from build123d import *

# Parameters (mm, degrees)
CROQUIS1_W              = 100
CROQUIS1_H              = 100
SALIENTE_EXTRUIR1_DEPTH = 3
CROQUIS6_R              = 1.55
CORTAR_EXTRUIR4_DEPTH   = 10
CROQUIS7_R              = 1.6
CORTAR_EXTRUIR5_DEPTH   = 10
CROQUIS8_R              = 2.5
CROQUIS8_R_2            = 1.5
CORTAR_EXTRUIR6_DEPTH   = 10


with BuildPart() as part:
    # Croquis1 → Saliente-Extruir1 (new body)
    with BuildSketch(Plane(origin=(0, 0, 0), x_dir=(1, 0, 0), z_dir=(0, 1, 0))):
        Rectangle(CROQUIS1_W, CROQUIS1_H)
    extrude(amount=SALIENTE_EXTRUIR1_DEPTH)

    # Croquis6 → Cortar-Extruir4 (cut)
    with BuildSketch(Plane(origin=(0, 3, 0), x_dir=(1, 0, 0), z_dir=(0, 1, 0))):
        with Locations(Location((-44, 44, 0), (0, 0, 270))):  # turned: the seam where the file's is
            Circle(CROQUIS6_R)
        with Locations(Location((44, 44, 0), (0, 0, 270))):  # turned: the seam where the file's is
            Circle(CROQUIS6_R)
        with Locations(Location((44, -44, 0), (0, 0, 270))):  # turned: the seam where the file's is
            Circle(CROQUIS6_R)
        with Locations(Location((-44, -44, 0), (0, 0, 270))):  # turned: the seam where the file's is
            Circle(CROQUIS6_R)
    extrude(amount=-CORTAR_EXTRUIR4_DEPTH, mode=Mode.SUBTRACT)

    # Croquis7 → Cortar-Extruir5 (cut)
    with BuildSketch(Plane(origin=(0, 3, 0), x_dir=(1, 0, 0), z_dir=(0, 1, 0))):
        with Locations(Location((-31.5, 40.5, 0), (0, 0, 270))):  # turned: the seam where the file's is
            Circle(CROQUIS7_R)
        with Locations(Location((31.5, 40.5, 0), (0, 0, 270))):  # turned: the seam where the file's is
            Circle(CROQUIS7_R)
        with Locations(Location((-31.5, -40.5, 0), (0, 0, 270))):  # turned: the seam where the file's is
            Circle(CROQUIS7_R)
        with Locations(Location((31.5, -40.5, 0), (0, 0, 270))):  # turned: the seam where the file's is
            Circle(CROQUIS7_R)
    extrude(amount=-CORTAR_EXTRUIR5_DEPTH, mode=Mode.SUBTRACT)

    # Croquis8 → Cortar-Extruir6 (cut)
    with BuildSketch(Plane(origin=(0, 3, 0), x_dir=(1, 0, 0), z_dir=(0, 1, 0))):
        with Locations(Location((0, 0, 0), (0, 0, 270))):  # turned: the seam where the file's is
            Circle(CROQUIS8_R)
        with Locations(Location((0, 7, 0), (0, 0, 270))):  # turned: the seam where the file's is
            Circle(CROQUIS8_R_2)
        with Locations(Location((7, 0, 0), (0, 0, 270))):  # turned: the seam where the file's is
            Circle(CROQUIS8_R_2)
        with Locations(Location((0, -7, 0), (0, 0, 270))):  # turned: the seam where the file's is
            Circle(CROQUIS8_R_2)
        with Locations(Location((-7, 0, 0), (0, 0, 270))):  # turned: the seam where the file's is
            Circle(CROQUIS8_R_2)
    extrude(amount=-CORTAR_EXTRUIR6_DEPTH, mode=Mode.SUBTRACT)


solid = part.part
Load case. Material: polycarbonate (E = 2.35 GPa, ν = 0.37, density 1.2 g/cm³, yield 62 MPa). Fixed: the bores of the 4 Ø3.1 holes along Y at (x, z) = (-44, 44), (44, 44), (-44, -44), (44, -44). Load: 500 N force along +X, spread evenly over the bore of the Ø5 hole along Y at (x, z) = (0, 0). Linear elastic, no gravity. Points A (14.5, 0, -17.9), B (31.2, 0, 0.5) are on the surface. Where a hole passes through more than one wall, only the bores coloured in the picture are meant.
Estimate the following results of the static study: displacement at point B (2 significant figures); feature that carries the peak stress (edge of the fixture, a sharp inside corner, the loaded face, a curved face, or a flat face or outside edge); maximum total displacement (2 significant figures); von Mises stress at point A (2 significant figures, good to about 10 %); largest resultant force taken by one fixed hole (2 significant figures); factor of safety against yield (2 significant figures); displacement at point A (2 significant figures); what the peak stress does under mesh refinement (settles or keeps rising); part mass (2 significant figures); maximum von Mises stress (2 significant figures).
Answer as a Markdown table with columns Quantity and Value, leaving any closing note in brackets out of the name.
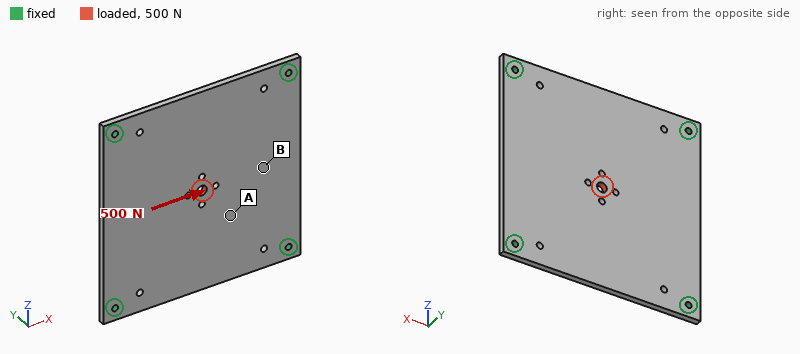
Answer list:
| Quantity | Value |
|---|---|
| displacement at point B | 0.058 mm |
| feature that carries the peak stress | a curved face |
| maximum total displacement | 0.11 mm |
| von Mises stress at point A | 2.1 MPa |
| largest resultant force taken by one fixed hole | 140 N |
| factor of safety against yield | 3.3 |
| displacement at point A | 0.050 mm |
| what the peak stress does under mesh refinement | settles |
| part mass | 36 g |
| maximum von Mises stress | 19 MPa |
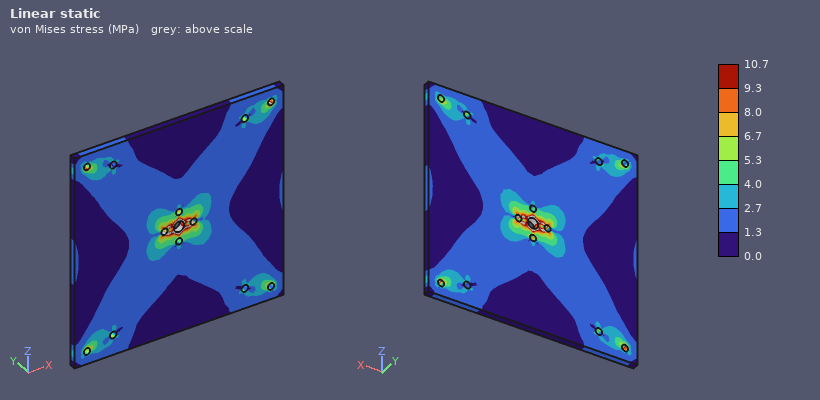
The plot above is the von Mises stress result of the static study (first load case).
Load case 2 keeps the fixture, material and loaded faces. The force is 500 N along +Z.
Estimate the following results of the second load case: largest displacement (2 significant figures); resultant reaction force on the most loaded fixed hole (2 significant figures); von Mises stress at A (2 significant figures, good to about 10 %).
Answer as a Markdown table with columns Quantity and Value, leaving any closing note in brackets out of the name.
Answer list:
| Quantity | Value |
|---|---|
| largest displacement | 0.11 mm |
| resultant reaction force on the most loaded fixed hole | 140 N |
| von Mises stress at A | 2.2 MPa |
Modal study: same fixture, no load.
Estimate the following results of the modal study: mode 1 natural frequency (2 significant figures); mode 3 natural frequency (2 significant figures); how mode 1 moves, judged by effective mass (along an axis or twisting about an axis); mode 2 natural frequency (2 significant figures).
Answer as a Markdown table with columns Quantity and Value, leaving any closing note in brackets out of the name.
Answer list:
| Quantity | Value |
|---|---|
| mode 1 natural frequency | 340 Hz |
| mode 3 natural frequency | 600 Hz |
| how mode 1 moves, judged by effective mass | along Y |
| mode 2 natural frequency | 600 Hz |
